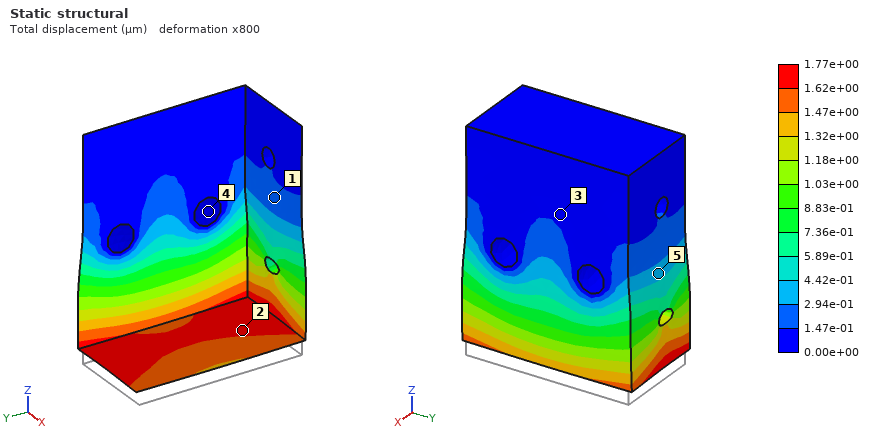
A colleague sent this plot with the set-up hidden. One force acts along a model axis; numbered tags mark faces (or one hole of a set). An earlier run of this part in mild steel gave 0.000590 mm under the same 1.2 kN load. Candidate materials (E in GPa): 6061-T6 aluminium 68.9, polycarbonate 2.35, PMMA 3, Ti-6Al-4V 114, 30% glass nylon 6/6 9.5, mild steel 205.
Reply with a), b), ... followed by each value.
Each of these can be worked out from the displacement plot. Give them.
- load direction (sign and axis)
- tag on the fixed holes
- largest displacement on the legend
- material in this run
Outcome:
a) +Z
b) 4
c) 1.77e+00 µm
d) 6061-T6 aluminium
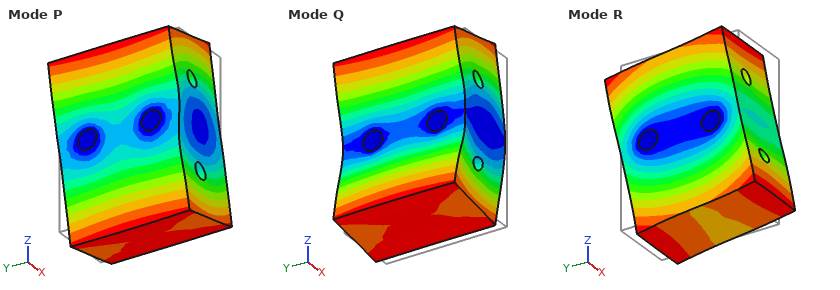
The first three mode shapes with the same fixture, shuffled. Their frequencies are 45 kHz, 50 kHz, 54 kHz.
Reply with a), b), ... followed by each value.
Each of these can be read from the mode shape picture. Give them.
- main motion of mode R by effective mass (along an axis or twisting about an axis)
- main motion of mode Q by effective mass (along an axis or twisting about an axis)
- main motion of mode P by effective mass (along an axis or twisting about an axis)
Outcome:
a) twisting about X
b) along X
c) twisting about Y
